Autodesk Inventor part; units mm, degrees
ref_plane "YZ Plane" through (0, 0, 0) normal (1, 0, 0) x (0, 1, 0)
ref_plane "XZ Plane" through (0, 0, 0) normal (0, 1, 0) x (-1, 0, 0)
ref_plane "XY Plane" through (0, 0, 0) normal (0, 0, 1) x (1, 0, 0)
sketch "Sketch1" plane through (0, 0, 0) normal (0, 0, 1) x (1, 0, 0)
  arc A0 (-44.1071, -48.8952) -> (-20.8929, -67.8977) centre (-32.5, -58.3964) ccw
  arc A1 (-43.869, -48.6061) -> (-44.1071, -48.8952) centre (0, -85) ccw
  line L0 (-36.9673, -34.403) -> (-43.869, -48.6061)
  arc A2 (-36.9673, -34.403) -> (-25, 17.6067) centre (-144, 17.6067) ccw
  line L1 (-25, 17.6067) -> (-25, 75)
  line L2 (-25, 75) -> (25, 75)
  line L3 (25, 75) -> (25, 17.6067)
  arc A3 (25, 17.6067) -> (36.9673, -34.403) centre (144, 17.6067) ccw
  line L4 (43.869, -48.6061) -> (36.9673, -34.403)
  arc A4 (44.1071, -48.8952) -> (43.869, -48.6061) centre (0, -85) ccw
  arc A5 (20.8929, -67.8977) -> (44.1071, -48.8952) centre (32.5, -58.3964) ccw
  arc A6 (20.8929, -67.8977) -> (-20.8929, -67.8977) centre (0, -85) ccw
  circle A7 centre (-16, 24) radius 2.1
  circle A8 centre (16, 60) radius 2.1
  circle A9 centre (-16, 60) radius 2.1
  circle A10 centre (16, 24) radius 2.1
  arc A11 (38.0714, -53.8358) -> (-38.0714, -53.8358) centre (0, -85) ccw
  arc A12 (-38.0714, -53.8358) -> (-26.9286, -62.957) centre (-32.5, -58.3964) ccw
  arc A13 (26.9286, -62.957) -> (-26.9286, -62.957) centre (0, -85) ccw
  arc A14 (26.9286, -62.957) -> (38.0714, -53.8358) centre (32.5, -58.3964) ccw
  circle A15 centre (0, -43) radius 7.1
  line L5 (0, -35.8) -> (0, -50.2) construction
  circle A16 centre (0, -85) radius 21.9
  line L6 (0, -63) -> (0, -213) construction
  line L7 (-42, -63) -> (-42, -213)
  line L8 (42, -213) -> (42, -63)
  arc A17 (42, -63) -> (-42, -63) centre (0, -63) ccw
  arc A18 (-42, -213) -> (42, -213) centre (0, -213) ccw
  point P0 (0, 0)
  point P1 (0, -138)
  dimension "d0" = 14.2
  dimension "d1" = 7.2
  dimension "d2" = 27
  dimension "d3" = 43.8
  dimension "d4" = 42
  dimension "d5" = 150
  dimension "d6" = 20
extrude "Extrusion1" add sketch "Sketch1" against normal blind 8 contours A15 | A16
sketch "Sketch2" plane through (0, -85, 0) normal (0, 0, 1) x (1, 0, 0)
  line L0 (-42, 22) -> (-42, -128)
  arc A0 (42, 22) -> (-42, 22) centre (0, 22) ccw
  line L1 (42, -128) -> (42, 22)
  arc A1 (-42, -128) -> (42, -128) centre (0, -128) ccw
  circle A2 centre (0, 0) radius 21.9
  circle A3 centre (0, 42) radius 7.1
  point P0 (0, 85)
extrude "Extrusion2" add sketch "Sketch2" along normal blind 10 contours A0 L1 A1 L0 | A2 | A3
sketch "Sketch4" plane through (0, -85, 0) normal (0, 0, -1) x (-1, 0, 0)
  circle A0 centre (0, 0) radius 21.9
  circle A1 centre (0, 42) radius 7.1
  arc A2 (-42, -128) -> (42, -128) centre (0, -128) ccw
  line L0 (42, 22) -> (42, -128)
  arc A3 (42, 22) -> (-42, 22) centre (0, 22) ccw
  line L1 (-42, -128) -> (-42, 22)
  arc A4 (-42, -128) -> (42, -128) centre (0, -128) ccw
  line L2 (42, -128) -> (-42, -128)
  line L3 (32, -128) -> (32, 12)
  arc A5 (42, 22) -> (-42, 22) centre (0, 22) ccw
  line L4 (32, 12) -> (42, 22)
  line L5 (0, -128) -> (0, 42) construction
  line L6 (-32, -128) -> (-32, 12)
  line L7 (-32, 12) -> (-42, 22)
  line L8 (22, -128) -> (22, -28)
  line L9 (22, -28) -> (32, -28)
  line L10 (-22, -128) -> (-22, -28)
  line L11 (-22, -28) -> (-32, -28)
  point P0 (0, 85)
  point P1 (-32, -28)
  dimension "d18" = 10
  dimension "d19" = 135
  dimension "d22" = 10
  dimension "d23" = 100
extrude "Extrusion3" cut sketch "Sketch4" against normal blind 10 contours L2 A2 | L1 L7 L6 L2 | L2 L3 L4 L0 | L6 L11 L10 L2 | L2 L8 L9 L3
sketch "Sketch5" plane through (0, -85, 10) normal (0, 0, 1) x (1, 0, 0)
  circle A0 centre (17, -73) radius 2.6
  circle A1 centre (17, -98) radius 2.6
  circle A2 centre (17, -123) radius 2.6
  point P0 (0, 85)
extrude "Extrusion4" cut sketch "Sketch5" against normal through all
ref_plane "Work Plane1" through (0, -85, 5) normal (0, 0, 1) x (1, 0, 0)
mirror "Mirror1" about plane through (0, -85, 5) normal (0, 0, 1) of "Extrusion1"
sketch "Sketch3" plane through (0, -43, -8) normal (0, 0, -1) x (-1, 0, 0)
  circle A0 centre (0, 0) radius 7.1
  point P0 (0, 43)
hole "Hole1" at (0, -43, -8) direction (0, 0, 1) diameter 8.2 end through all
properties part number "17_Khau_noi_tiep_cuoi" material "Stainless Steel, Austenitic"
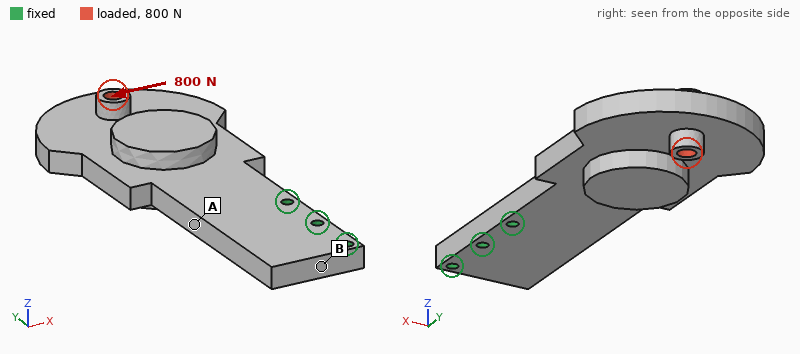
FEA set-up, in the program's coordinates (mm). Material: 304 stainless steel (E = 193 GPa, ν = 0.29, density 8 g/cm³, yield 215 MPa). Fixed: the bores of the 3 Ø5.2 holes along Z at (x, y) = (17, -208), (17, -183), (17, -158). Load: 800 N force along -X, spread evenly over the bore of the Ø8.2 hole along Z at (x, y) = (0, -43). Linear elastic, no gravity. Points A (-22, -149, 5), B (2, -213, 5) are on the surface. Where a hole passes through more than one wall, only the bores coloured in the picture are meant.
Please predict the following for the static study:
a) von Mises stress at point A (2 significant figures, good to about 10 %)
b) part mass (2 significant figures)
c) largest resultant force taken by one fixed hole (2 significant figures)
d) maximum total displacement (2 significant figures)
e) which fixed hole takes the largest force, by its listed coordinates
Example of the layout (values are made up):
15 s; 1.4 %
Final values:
25 MPa; 1.0 kg; 3.3 kN; 53 µm; (17, -158)
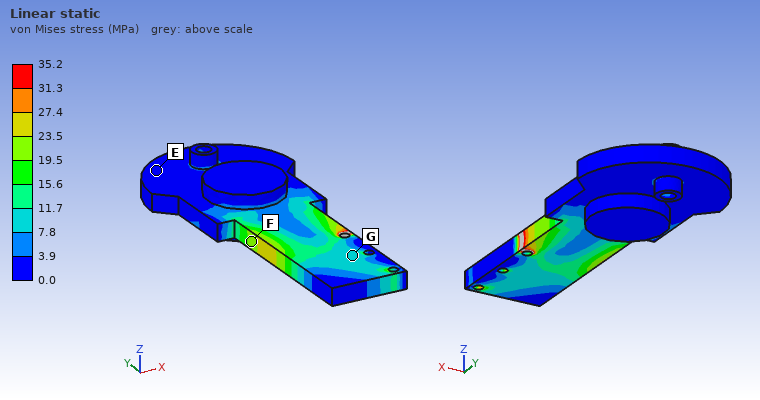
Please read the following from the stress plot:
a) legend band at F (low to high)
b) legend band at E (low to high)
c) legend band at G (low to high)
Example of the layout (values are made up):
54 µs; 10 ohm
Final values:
19.5 to 23.5 MPa; 0.0 to 3.9 MPa; 7.8 to 11.7 MPa
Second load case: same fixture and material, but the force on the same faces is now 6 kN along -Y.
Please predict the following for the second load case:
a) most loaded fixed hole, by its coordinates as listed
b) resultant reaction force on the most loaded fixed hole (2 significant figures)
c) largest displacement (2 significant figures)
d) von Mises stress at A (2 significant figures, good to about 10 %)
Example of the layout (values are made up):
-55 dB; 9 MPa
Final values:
(17, -158); 3.8 kN; 22 µm; 17 MPa
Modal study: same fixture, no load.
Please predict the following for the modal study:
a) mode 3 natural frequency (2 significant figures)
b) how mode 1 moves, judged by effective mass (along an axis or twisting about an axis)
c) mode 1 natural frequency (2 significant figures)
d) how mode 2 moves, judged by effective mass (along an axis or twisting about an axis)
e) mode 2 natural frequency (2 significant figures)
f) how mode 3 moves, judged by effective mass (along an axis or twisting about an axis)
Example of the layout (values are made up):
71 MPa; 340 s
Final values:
1200 Hz; along Z; 300 Hz; along X; 1100 Hz; twisting about Y
